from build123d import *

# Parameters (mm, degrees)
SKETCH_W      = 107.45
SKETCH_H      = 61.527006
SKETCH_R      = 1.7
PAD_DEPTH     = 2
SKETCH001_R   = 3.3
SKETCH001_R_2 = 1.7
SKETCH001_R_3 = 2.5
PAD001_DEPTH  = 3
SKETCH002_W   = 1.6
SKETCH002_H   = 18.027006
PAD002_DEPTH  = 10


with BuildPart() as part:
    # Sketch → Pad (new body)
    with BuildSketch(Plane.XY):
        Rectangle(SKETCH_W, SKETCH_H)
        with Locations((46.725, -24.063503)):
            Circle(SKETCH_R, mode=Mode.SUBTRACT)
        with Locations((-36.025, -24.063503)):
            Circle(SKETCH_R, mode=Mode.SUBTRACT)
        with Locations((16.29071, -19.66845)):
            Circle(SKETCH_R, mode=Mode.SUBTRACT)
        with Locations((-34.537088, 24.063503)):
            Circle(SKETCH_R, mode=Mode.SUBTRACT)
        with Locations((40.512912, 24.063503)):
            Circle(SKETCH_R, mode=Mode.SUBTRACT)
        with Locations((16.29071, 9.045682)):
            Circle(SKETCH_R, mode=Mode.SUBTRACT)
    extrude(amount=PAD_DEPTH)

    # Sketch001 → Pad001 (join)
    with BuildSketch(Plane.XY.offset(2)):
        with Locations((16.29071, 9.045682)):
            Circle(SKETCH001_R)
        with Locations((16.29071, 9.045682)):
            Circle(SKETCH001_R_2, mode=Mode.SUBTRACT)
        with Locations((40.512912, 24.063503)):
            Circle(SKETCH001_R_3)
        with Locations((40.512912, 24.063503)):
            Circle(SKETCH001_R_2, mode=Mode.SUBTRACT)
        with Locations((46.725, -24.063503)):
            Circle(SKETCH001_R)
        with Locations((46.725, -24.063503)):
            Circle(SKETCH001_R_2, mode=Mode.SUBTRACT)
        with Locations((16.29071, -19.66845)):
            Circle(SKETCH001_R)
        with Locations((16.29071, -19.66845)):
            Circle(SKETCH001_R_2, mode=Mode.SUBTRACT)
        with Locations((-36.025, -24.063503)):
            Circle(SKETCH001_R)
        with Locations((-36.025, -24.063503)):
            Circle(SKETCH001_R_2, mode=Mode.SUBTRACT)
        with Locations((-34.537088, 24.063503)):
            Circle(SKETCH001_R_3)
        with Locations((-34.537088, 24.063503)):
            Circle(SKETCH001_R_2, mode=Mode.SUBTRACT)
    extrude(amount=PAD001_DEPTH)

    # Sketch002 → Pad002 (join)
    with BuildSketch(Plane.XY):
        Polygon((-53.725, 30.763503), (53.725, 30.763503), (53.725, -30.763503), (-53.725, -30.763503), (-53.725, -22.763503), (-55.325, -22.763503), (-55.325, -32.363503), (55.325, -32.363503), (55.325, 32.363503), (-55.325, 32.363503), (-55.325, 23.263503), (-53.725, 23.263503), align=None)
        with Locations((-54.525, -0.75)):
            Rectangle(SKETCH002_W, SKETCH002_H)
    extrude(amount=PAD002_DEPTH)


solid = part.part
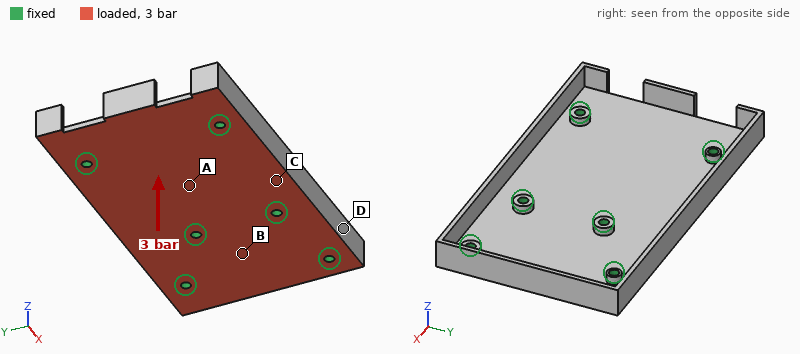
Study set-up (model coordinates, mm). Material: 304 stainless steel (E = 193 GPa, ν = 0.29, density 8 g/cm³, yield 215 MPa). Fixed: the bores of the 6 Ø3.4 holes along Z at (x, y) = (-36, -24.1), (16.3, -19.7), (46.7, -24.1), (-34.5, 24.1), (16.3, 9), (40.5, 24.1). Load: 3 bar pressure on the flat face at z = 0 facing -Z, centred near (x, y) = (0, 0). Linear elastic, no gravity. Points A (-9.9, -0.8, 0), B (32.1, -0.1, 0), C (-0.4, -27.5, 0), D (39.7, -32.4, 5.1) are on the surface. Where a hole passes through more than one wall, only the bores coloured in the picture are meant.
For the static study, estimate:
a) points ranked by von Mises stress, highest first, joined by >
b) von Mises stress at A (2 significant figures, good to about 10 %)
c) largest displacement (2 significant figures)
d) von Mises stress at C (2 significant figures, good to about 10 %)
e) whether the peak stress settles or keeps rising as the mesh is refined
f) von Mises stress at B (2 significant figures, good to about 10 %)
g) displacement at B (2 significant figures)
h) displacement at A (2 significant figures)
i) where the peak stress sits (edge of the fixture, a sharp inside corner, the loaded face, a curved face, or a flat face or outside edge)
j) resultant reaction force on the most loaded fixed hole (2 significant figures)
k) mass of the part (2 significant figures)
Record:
A > C > B > D
40 MPa
52 µm
30 MPa
keeps rising
16 MPa
11 µm
49 µm
edge of the fixture
470 N
150 g
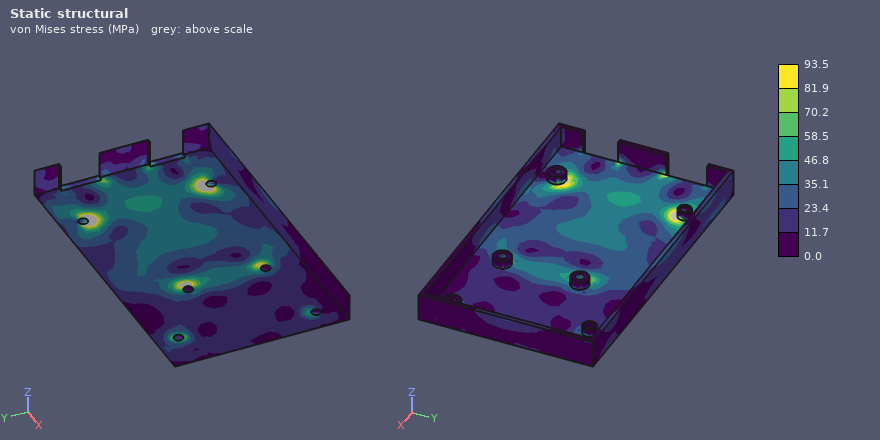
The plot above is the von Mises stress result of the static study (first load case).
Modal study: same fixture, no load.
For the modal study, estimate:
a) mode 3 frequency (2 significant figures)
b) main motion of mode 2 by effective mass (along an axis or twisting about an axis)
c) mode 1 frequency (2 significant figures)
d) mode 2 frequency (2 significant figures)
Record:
4600 Hz
along Z
3000 Hz
3700 Hz
